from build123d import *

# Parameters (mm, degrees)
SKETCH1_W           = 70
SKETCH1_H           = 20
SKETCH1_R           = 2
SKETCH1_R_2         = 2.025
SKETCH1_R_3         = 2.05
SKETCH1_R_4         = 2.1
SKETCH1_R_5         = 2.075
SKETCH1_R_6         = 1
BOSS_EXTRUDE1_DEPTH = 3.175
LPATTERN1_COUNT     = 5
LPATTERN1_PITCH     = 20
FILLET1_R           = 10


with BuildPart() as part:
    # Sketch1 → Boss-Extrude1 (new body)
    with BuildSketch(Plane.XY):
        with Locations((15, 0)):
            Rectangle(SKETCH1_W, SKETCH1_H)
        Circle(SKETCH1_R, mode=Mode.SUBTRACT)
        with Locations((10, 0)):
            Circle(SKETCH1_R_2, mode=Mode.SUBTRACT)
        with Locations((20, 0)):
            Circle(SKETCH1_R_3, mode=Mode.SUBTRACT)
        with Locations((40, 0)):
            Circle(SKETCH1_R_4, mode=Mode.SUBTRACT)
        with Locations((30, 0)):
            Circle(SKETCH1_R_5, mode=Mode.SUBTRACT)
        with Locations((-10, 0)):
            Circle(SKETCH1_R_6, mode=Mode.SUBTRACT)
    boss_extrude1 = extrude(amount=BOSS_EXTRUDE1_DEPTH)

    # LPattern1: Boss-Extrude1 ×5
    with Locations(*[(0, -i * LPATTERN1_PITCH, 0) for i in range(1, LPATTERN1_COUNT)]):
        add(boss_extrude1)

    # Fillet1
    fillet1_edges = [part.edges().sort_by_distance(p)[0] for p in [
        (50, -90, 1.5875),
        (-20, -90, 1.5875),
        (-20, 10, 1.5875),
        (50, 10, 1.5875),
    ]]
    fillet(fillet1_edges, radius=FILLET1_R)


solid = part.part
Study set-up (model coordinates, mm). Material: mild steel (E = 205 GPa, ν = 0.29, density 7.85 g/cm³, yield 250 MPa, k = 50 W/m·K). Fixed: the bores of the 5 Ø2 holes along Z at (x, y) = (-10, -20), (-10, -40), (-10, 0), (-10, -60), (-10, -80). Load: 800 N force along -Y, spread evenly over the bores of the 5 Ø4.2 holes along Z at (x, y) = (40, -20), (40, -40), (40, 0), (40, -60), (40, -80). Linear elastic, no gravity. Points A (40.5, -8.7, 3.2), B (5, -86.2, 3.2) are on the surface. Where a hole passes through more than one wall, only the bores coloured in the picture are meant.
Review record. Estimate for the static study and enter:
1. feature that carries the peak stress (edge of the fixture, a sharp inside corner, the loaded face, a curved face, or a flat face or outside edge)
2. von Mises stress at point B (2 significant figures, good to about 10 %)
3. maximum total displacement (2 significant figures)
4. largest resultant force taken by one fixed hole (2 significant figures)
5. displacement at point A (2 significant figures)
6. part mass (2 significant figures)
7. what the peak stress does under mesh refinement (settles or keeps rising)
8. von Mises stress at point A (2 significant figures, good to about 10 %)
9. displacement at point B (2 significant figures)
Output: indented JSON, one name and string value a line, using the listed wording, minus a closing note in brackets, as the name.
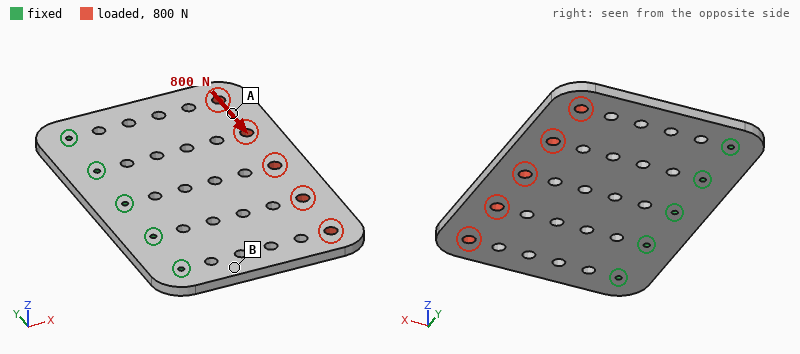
{
  "feature that carries the peak stress": "edge of the fixture",
  "von Mises stress at point B": "6.1 MPa",
  "maximum total displacement": "4.1 µm",
  "largest resultant force taken by one fixed hole": "460 N",
  "displacement at point A": "3.5 µm",
  "part mass": "160 g",
  "what the peak stress does under mesh refinement": "keeps rising",
  "von Mises stress at point A": "2.2 MPa",
  "displacement at point B": "1.5 µm"
}
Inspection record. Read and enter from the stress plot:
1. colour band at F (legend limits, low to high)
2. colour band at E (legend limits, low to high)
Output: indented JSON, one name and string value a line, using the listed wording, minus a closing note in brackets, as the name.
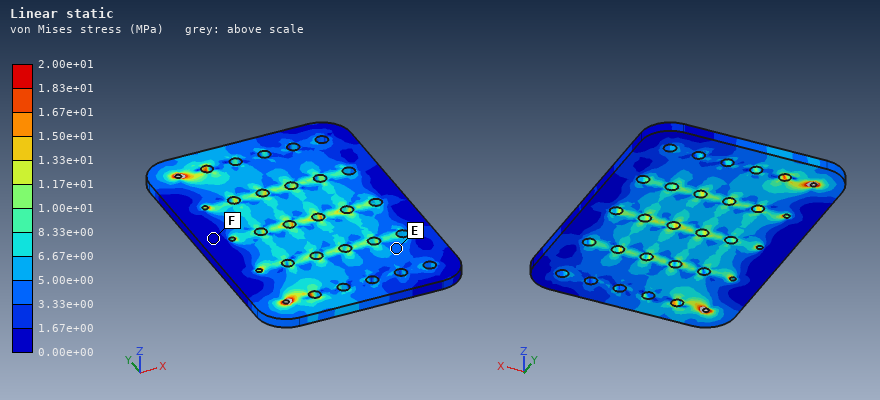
{
  "colour band at F": "0.00e+00 to 1.67e+00 MPa",
  "colour band at E": "3.33e+00 to 5.00e+00 MPa"
}
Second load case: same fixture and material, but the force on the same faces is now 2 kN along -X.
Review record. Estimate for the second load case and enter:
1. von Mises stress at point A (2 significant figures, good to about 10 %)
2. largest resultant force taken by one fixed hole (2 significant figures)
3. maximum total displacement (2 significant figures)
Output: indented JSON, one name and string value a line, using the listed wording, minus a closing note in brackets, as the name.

{
  "von Mises stress at point A": "3.9 MPa",
  "largest resultant force taken by one fixed hole": "430 N",
  "maximum total displacement": "2.3 µm"
}
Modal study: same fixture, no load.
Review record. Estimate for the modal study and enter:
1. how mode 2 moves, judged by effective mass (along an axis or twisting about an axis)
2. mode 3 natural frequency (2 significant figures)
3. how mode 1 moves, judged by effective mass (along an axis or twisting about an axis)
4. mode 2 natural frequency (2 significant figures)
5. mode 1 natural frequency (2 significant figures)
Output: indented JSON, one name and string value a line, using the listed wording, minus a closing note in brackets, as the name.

{
  "how mode 2 moves, judged by effective mass": "twisting about X",
  "mode 3 natural frequency": "2600 Hz",
  "how mode 1 moves, judged by effective mass": "along Z",
  "mode 2 natural frequency": "1200 Hz",
  "mode 1 natural frequency": "690 Hz"
}
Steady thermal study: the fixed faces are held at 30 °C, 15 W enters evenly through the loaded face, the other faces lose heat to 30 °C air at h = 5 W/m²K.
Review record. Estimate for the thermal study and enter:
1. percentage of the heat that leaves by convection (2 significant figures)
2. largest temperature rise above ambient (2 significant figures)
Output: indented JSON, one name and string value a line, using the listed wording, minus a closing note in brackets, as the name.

{
  "percentage of the heat that leaves by convection": "13 %",
  "largest temperature rise above ambient": "54 K"
}
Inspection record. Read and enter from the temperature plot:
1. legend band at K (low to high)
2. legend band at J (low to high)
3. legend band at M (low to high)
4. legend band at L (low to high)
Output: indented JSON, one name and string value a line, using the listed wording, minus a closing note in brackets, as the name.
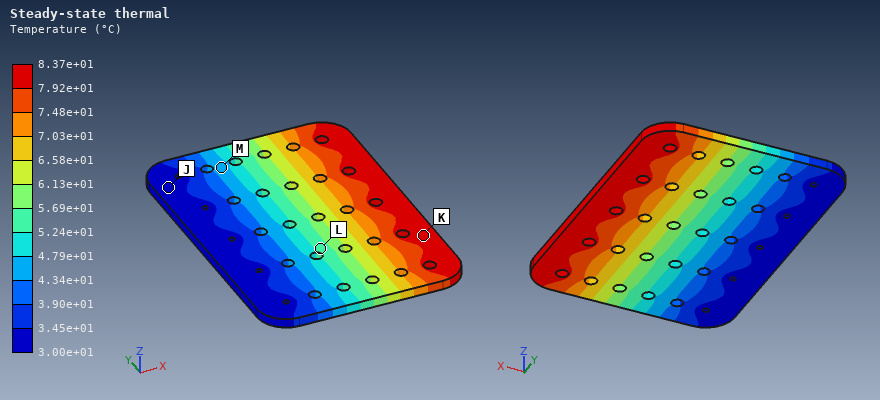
{
  "legend band at K": "7.92e+01 to 8.37e+01 °C",
  "legend band at J": "3.00e+01 to 3.45e+01 °C",
  "legend band at M": "4.34e+01 to 4.79e+01 °C",
  "legend band at L": "5.24e+01 to 5.69e+01 °C"
}
